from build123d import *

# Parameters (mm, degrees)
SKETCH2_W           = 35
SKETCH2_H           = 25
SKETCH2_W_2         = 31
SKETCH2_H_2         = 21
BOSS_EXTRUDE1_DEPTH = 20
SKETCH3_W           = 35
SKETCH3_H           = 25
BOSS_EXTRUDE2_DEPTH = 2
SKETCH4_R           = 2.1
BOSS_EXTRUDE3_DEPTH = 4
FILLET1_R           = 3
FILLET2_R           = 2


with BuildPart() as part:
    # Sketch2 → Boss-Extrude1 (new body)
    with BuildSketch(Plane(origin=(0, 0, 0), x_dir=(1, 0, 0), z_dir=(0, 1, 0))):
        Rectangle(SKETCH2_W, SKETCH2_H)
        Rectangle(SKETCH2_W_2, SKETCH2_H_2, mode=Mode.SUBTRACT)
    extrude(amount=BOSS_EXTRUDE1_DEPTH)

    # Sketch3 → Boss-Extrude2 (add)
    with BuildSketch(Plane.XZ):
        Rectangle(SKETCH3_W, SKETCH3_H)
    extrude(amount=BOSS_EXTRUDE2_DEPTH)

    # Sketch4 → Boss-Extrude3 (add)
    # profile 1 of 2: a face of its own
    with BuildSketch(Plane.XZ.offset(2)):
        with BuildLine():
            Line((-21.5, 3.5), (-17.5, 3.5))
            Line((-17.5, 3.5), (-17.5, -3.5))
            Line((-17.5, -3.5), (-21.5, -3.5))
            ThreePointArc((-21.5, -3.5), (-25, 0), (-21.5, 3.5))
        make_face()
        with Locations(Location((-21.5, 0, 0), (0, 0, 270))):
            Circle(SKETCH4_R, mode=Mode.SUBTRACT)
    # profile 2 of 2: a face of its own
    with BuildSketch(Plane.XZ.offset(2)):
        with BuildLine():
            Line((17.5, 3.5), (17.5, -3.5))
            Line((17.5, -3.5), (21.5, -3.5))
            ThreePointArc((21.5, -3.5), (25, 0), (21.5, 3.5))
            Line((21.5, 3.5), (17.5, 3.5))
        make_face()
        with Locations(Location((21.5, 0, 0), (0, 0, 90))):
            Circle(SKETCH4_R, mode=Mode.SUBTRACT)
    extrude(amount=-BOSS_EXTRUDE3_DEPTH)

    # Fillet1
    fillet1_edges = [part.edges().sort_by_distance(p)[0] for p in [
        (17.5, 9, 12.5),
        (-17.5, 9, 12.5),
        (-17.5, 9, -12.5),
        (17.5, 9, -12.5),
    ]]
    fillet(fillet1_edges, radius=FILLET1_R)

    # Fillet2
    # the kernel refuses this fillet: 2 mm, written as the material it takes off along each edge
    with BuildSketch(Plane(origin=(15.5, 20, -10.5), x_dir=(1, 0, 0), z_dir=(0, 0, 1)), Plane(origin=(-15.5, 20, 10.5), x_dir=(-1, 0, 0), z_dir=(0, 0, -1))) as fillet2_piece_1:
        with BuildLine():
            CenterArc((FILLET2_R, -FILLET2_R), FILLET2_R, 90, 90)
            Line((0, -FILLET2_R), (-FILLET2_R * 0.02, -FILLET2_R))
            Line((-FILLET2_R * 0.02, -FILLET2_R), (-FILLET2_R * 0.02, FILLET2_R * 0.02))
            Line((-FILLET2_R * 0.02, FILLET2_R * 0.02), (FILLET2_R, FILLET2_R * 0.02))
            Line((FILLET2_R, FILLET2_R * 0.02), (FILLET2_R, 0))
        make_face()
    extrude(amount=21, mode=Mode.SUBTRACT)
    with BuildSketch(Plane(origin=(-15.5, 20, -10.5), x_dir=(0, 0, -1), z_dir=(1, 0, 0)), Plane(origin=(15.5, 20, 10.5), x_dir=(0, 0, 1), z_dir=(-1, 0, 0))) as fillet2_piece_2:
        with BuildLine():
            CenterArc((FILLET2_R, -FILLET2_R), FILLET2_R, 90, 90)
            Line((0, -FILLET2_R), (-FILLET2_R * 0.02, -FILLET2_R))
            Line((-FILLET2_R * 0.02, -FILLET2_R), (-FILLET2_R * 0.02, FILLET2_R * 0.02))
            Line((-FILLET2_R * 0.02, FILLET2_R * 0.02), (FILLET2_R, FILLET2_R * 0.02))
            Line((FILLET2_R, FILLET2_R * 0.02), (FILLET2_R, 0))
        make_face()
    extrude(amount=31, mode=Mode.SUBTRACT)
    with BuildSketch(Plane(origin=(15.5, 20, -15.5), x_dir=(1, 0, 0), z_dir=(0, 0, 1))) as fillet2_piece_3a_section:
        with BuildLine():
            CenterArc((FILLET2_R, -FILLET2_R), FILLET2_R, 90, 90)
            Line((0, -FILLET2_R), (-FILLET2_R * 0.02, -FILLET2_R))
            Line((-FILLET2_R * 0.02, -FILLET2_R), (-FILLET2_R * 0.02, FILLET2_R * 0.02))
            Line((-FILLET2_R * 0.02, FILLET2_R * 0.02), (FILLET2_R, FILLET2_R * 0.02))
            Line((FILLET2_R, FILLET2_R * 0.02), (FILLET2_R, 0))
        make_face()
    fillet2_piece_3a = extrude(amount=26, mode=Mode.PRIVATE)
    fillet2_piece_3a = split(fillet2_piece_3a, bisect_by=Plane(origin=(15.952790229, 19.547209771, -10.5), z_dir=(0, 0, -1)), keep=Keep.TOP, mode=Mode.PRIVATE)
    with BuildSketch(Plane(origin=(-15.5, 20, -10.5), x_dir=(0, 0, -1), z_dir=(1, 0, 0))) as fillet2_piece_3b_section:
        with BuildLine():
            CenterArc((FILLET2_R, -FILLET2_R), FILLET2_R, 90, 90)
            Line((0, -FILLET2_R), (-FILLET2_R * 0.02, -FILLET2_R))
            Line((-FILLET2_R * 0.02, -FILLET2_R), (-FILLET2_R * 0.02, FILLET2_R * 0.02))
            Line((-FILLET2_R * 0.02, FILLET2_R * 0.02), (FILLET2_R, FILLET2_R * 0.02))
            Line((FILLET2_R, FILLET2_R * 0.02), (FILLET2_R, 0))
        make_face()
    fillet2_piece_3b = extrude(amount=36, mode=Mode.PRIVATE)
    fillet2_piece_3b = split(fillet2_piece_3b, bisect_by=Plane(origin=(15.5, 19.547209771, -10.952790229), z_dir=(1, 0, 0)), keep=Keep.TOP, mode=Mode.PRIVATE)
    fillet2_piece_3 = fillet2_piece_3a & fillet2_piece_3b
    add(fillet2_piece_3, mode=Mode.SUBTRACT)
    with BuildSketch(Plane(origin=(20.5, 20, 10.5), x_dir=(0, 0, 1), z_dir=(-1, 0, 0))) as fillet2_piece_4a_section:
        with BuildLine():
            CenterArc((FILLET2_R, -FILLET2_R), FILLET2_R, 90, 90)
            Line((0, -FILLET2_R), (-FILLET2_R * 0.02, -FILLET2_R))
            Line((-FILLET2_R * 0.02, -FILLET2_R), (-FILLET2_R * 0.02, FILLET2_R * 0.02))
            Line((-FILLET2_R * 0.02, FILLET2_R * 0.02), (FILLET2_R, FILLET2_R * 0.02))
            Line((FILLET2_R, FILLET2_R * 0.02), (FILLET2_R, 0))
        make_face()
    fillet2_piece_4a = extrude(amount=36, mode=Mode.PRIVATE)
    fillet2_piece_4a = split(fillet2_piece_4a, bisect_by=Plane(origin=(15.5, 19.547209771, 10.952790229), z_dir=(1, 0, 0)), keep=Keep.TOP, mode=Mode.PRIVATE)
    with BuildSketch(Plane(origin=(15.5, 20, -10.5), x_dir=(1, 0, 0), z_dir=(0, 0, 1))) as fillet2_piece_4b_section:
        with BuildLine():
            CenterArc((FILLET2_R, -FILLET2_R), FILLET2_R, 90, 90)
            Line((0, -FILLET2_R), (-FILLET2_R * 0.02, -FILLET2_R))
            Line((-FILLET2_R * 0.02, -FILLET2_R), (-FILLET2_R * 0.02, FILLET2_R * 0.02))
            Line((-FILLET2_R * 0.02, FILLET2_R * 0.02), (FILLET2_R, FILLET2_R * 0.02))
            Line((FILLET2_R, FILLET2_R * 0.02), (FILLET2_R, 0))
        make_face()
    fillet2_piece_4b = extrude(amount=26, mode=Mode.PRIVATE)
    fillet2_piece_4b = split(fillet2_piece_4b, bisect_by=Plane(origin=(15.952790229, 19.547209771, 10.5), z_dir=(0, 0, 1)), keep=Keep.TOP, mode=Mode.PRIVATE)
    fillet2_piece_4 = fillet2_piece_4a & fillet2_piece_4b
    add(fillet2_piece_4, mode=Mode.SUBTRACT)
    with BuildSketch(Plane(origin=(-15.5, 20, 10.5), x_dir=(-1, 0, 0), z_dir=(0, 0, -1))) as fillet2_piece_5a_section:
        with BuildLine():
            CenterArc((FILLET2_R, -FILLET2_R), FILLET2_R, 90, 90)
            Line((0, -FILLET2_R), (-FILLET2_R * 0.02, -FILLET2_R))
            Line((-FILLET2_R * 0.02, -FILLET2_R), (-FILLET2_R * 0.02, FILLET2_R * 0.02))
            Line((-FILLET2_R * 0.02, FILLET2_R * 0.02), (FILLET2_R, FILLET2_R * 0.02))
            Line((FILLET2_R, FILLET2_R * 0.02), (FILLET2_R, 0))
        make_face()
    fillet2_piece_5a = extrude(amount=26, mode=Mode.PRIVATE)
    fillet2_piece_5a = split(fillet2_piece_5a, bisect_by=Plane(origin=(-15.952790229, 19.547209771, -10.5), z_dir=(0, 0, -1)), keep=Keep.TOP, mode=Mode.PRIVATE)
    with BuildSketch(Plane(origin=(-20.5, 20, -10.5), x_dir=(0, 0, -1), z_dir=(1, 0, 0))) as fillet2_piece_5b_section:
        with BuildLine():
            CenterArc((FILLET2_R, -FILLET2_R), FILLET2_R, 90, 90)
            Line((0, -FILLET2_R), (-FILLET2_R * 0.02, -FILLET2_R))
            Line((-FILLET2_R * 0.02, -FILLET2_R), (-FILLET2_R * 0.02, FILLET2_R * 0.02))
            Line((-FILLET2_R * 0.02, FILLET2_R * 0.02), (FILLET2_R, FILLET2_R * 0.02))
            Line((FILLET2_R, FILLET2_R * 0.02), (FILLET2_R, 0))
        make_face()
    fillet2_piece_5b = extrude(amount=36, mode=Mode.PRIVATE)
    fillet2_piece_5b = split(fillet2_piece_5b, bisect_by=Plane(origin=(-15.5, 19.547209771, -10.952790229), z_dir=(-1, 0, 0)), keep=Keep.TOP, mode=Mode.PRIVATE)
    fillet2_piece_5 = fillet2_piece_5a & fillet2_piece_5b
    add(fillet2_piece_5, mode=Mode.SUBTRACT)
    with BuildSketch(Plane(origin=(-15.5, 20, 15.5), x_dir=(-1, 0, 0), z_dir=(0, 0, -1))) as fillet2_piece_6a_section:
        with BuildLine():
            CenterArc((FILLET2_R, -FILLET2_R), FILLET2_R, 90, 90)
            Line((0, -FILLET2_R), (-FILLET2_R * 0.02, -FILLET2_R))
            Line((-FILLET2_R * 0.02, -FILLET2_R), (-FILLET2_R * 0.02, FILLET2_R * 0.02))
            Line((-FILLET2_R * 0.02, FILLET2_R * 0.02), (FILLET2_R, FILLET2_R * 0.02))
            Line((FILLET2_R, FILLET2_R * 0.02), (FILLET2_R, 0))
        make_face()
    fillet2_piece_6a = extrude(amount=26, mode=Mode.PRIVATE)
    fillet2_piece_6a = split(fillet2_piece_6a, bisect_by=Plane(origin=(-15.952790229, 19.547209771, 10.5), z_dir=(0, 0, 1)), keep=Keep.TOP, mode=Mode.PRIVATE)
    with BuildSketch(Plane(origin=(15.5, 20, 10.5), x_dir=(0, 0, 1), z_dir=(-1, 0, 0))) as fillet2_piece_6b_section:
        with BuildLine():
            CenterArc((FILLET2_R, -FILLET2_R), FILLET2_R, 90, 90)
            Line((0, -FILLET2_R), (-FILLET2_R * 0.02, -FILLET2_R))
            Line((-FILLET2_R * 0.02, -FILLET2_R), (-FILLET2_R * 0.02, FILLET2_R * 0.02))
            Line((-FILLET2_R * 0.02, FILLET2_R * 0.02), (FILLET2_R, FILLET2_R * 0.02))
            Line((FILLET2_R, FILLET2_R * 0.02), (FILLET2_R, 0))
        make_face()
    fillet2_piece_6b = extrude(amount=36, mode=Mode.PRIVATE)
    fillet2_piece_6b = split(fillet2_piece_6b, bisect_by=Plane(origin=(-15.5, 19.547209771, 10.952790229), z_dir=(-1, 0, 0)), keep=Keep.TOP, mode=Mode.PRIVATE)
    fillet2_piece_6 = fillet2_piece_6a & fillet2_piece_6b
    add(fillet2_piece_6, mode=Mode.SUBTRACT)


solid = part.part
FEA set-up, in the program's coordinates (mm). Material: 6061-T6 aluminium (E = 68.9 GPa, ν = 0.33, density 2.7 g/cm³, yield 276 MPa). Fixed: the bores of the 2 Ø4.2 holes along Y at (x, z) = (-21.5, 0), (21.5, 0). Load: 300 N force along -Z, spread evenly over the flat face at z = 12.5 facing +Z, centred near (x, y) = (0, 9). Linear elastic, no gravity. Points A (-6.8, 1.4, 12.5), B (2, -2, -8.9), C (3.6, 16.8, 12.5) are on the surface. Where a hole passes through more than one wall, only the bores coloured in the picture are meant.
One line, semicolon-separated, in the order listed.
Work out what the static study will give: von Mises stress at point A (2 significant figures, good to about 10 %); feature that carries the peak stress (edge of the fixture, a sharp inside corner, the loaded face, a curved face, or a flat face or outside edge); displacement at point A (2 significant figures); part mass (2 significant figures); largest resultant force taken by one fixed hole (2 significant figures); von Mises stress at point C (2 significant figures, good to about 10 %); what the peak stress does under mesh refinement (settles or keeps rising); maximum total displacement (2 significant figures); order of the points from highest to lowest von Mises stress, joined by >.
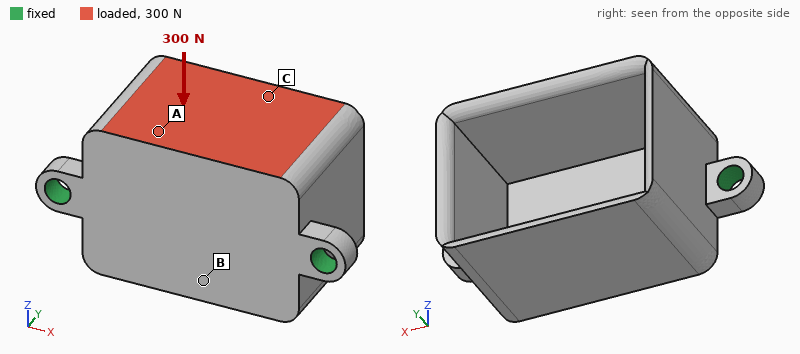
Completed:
18 MPa; edge of the fixture; 27 µm; 17 g; 150 N; 30 MPa; keeps rising; 99 µm; C > A > B
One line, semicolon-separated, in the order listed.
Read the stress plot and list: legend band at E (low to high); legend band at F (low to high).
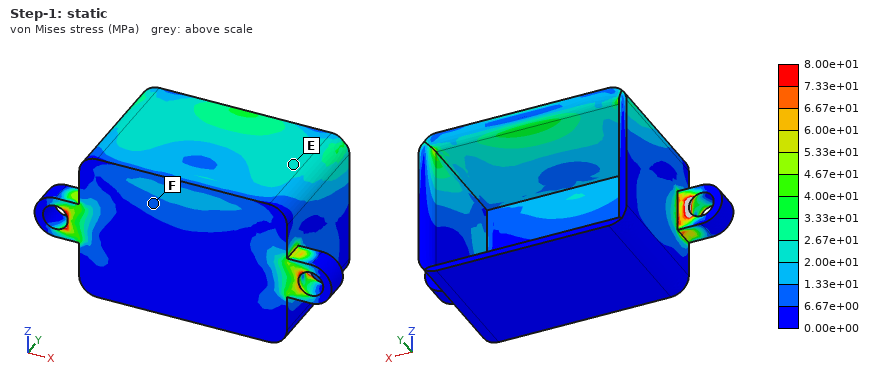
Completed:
2.00e+01 to 2.67e+01 MPa; 6.67e+00 to 1.33e+01 MPa
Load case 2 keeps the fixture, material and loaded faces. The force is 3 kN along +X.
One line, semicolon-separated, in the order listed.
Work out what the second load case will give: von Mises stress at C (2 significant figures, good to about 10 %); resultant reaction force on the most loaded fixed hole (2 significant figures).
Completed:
41 MPa; 1.9 kN
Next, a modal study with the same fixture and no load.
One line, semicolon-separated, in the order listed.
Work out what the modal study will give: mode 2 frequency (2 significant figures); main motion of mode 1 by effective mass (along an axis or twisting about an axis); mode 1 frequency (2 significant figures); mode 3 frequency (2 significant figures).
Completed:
6100 Hz; along Z; 3600 Hz; 7900 Hz
